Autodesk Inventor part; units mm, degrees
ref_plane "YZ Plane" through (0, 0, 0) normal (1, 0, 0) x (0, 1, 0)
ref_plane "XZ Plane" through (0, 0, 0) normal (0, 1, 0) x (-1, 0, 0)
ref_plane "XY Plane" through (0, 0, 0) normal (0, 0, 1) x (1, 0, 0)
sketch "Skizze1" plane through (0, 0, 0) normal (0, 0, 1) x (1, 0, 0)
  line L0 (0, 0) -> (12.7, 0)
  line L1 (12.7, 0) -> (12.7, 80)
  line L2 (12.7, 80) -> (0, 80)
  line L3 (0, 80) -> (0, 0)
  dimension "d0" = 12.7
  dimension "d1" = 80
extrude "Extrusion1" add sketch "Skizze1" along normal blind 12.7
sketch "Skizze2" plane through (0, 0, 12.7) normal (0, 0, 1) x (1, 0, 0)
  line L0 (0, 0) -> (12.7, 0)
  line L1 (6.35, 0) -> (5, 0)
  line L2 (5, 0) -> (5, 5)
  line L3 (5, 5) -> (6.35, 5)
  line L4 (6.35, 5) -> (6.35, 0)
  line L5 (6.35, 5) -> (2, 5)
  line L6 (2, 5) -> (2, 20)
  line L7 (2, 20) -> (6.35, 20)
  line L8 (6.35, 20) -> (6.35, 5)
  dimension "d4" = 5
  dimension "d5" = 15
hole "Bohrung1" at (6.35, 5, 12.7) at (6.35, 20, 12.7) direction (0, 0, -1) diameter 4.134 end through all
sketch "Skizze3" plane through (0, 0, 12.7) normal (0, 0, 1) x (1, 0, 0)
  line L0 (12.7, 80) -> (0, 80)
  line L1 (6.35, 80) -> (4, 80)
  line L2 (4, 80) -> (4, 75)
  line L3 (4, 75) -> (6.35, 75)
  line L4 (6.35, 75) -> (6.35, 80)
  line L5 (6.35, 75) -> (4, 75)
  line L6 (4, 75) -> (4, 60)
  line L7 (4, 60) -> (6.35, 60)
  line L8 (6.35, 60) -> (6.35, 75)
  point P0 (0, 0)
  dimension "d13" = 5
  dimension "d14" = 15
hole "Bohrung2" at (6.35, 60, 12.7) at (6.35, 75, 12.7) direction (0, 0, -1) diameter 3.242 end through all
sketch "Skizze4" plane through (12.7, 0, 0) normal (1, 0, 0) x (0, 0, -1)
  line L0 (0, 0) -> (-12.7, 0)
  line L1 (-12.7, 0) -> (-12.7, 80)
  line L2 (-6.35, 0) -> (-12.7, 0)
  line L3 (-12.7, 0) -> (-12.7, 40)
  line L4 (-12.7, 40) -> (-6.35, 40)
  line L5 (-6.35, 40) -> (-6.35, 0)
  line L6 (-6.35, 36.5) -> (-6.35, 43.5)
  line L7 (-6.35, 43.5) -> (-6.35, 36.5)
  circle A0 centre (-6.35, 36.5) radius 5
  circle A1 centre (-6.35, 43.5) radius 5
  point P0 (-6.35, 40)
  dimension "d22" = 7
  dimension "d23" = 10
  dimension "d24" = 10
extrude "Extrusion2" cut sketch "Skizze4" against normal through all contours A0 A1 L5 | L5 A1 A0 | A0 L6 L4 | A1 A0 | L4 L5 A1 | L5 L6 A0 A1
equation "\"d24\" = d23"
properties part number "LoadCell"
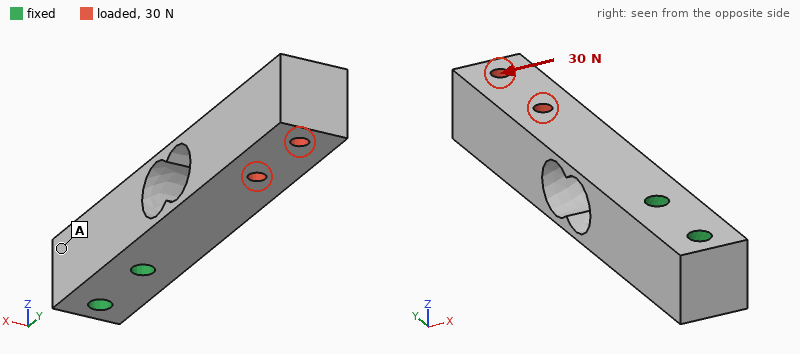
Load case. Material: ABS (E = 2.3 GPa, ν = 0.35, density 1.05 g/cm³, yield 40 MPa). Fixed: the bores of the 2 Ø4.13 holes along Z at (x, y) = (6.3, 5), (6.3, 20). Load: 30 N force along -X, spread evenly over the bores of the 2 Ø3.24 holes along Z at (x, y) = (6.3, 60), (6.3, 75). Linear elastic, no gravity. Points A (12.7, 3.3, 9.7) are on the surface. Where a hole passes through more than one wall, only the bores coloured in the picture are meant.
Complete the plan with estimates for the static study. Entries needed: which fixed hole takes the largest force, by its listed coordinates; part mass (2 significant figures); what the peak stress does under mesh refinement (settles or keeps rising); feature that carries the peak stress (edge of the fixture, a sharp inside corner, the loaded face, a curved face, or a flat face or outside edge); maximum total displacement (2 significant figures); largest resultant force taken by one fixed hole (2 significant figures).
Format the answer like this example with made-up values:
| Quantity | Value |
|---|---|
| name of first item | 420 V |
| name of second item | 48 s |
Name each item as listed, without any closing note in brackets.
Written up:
| Quantity | Value |
|---|---|
| which fixed hole takes the largest force, by its listed coordinates | (6.3, 20) |
| part mass | 11 g |
| what the peak stress does under mesh refinement | keeps rising |
| feature that carries the peak stress | a sharp inside corner |
| maximum total displacement | 0.80 mm |
| largest resultant force taken by one fixed hole | 75 N |
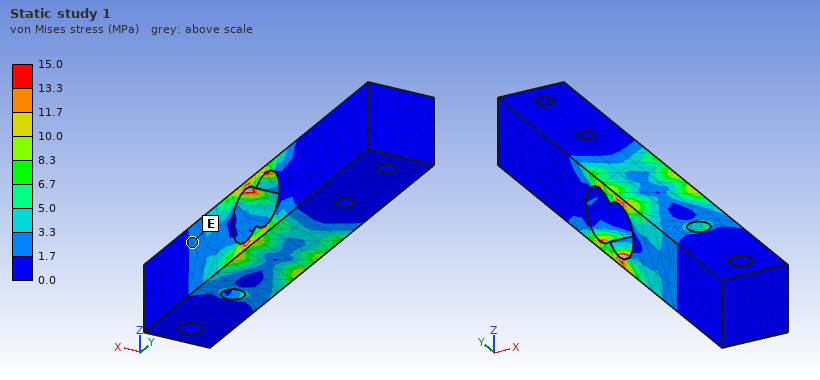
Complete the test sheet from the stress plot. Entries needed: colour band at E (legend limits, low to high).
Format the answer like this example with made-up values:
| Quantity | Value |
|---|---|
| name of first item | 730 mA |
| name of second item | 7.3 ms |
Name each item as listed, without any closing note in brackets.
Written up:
| Quantity | Value |
|---|---|
| colour band at E | 1.7 to 3.3 MPa |
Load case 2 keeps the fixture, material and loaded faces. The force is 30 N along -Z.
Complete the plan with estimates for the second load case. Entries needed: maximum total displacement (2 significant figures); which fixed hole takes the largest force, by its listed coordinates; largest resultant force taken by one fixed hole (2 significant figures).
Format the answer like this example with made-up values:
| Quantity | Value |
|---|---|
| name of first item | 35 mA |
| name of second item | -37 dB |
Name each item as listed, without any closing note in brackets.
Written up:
| Quantity | Value |
|---|---|
| maximum total displacement | 0.75 mm |
| which fixed hole takes the largest force, by its listed coordinates | (6.3, 20) |
| largest resultant force taken by one fixed hole | 42 N |
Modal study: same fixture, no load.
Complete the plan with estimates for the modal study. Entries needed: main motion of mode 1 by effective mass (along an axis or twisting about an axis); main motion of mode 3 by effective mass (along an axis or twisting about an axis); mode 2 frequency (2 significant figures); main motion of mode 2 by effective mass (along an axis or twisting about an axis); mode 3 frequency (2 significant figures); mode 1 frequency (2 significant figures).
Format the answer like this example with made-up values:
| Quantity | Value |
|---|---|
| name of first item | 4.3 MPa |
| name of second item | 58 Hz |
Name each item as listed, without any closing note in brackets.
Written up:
| Quantity | Value |
|---|---|
| main motion of mode 1 by effective mass | along Z |
| main motion of mode 3 by effective mass | twisting about Y |
| mode 2 frequency | 540 Hz |
| main motion of mode 2 by effective mass | along X |
| mode 3 frequency | 2000 Hz |
| mode 1 frequency | 490 Hz |
